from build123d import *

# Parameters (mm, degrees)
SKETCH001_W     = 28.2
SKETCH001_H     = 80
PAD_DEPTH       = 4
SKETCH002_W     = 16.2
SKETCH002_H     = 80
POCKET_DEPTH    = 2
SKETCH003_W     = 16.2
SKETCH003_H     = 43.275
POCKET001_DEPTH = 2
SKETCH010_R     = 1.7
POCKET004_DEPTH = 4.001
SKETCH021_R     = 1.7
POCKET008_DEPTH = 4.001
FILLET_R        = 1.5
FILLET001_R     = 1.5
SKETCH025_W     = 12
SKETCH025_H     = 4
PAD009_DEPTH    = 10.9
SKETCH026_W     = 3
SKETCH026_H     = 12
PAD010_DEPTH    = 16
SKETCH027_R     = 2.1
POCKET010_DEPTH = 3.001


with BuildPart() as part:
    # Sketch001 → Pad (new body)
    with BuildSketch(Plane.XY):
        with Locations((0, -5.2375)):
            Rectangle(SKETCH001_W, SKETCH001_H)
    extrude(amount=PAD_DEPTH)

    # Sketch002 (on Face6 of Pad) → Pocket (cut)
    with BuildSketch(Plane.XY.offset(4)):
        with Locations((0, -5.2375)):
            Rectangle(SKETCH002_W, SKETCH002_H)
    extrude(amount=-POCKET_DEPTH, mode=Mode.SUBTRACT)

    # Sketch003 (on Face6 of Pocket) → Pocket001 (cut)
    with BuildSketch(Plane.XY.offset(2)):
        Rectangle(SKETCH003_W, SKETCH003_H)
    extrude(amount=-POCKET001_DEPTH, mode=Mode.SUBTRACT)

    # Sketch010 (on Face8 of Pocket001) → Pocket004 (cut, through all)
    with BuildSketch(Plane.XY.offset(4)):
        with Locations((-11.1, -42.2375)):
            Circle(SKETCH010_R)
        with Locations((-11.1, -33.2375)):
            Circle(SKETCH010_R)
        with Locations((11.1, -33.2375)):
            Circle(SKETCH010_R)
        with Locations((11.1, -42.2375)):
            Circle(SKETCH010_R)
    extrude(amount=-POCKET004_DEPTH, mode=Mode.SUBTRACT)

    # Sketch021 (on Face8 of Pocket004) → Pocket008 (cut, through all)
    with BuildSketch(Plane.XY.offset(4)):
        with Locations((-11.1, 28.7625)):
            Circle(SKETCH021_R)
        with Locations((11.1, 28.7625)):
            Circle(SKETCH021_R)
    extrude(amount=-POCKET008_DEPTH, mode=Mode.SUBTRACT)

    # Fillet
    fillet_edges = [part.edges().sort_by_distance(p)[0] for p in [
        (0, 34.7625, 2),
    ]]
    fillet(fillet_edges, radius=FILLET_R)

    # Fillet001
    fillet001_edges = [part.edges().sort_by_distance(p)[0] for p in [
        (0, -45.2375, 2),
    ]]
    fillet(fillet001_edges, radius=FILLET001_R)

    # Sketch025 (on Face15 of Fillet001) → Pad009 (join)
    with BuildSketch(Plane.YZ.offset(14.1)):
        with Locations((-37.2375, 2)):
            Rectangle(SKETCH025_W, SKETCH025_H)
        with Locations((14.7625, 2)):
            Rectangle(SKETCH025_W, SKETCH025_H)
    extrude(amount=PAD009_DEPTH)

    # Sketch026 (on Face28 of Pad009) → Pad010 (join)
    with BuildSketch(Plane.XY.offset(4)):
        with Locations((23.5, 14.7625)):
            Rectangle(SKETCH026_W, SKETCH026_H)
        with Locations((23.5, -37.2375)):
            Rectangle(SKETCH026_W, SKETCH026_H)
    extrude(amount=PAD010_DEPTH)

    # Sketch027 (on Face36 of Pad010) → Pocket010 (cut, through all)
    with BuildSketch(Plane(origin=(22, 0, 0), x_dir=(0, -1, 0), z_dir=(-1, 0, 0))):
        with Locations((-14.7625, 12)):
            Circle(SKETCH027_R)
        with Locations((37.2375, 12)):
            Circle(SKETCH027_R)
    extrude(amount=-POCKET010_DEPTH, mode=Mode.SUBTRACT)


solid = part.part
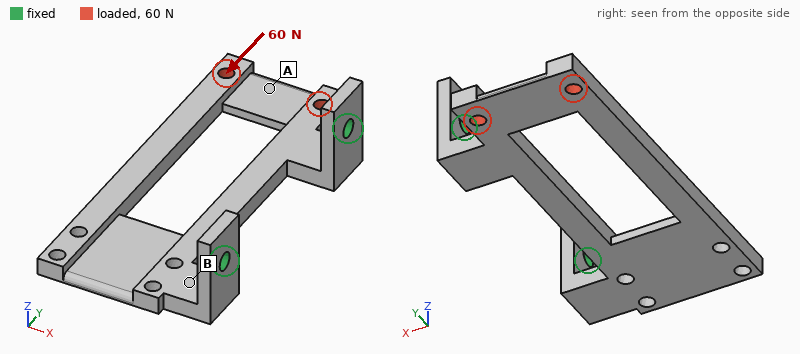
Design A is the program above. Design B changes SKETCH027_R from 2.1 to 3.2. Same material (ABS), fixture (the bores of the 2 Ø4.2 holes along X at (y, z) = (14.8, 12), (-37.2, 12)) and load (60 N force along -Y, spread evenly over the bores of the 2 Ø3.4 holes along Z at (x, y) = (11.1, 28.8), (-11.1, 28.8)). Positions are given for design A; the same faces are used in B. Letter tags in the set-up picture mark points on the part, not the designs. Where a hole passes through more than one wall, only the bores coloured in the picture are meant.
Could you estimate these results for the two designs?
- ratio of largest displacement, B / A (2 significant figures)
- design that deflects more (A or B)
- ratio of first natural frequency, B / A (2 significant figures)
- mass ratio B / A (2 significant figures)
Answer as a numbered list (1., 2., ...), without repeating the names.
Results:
1. 0.86
2. A
3. 1.0
4. 0.98
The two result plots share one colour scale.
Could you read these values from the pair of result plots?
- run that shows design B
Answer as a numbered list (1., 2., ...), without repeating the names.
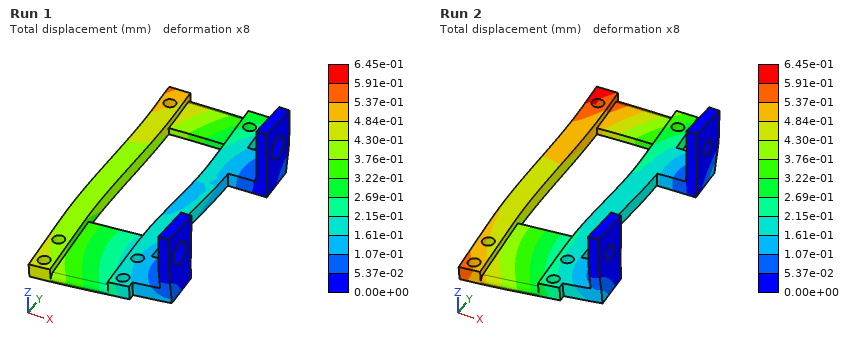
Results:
1. Run 1
